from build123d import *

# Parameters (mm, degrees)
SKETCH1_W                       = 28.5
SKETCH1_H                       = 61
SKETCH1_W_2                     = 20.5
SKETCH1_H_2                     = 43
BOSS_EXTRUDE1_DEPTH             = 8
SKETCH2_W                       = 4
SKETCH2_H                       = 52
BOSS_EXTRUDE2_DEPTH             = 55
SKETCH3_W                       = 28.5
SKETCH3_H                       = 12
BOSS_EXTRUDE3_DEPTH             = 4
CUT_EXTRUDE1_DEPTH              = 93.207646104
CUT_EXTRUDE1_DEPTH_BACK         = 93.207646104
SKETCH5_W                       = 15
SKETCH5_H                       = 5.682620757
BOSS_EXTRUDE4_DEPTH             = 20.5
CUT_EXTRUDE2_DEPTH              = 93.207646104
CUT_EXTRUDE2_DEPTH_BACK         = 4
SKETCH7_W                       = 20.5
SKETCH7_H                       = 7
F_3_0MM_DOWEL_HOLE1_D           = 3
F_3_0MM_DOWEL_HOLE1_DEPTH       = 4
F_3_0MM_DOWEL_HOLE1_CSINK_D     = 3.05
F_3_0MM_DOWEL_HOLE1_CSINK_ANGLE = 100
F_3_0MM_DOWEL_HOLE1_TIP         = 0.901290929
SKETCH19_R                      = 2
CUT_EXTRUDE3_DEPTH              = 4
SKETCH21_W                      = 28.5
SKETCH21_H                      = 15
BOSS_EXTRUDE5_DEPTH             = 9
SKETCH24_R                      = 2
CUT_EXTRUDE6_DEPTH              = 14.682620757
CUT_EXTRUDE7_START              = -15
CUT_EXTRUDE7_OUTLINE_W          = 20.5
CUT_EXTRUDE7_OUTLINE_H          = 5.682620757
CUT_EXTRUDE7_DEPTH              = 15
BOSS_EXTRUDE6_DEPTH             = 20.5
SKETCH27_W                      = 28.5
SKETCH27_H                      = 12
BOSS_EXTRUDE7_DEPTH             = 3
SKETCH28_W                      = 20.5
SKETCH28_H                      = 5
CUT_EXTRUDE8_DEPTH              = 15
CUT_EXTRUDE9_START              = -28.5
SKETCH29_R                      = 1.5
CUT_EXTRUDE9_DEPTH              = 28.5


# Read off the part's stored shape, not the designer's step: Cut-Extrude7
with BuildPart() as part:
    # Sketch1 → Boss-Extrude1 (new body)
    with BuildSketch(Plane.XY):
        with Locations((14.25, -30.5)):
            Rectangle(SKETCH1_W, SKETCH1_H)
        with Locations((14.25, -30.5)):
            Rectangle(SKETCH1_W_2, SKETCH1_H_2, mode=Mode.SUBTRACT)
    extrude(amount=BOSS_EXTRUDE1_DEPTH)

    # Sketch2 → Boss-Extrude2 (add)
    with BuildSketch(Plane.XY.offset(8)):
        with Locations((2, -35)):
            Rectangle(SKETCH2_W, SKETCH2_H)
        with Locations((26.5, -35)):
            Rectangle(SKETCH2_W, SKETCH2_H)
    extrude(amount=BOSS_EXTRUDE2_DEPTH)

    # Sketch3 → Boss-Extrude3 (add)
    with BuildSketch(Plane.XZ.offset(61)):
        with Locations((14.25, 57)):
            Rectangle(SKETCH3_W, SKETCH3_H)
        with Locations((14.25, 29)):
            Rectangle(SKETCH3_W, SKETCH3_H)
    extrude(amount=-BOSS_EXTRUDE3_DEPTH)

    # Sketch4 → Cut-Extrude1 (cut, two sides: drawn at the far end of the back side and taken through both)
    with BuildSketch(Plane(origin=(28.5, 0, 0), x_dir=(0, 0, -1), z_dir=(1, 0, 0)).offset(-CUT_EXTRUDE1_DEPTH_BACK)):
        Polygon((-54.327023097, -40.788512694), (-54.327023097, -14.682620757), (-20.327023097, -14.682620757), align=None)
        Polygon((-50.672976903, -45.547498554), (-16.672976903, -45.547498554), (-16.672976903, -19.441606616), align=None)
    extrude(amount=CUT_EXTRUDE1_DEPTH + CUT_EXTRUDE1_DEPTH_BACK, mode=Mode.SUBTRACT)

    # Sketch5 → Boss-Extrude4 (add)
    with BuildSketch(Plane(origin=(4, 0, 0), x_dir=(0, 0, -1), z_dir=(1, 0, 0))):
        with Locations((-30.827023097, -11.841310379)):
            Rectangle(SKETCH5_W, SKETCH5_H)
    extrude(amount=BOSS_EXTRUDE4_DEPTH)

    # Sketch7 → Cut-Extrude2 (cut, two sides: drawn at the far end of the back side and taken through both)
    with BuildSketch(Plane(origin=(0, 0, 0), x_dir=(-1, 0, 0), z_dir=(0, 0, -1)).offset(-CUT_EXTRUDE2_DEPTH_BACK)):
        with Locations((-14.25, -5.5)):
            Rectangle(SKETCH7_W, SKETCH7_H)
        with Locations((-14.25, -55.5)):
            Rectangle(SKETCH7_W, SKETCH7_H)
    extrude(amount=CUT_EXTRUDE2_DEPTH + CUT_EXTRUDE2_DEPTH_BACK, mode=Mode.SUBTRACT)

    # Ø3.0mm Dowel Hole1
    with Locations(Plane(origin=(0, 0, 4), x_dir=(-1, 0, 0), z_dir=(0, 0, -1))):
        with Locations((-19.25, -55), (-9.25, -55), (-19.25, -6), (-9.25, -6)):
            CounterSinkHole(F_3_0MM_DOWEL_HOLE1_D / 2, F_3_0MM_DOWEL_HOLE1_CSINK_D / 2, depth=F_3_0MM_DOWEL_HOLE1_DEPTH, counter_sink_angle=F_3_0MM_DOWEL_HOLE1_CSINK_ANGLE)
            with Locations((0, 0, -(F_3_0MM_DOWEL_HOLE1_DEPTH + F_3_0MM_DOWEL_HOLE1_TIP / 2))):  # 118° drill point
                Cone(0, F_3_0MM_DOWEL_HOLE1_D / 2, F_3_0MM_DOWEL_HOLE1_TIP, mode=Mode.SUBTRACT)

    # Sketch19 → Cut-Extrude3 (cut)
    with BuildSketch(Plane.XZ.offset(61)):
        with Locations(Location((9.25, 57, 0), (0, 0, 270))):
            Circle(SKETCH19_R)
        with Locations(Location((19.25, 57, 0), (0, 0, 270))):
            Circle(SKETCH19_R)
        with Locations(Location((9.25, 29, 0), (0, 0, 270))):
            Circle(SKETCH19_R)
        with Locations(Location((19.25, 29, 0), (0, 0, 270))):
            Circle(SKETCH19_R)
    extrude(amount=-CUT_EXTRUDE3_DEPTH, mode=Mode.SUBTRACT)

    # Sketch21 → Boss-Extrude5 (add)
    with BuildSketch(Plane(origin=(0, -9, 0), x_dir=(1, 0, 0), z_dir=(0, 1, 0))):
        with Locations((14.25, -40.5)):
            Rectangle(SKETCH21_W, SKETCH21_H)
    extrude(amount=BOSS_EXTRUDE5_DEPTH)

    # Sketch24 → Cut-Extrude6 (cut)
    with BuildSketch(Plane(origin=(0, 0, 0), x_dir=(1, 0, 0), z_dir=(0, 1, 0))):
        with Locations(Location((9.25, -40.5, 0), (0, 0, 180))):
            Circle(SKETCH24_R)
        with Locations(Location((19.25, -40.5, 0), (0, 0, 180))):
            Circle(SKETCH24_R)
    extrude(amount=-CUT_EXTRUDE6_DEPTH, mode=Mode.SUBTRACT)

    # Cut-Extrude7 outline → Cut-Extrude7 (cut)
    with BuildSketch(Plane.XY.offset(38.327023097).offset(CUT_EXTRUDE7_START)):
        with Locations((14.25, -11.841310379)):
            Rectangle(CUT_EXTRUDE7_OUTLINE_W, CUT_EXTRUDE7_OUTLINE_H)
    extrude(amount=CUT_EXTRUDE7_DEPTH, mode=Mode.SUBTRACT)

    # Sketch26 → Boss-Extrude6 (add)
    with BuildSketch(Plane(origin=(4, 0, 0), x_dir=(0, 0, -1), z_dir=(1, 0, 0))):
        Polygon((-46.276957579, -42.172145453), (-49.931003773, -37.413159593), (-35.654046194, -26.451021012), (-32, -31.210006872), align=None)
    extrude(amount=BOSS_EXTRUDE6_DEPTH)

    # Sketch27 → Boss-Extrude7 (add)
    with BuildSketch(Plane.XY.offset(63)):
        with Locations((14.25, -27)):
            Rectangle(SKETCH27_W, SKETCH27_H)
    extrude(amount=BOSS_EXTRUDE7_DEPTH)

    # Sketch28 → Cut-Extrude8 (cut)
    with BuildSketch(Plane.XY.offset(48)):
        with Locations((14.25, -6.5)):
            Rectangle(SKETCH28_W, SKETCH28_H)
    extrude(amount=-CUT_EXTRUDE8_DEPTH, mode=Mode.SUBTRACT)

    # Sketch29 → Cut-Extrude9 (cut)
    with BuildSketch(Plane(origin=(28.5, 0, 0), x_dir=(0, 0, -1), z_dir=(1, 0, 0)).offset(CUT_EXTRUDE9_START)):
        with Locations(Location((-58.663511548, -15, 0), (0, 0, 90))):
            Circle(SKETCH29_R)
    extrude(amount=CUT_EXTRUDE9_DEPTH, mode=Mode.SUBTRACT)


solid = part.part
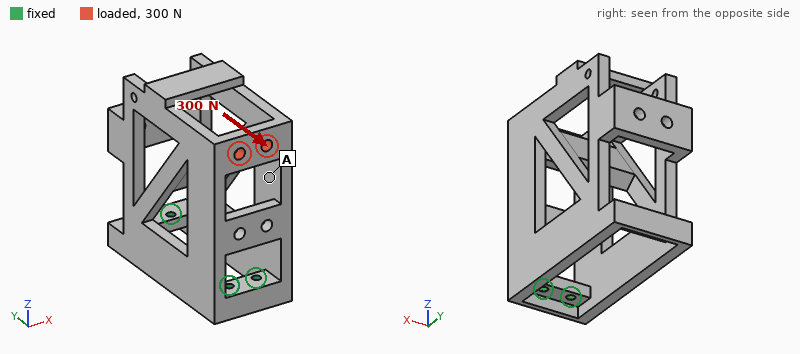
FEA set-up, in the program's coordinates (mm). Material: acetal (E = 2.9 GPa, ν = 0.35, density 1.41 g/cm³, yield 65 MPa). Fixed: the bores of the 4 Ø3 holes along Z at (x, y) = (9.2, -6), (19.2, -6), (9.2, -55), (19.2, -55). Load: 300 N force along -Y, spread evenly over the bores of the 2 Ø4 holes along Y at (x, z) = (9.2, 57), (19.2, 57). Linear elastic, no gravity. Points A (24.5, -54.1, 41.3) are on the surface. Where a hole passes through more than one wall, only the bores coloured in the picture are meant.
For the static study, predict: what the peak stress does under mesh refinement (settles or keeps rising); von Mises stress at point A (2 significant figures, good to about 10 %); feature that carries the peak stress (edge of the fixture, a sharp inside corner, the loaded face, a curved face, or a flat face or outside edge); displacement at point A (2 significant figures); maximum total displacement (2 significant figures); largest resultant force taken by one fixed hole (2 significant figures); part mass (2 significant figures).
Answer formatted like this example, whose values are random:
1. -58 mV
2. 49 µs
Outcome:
1. keeps rising
2. 4.1 MPa
3. edge of the fixture
4. 0.32 mm
5. 0.68 mm
6. 180 N
7. 40 g
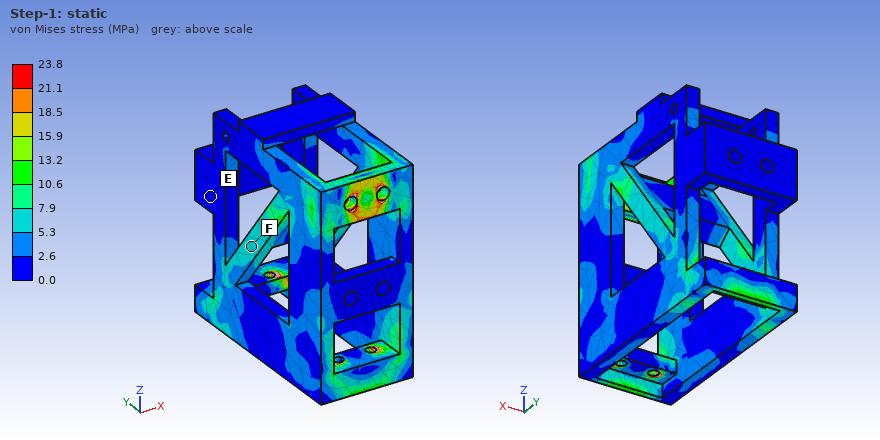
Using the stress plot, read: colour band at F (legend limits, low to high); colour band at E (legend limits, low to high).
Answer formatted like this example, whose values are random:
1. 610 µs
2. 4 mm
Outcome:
1. 5.3 to 7.9 MPa
2. 0.0 to 2.6 MPa
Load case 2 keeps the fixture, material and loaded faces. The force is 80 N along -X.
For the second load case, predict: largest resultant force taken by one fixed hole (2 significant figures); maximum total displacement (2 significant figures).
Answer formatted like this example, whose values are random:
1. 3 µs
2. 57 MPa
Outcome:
1. 140 N
2. 0.94 mm
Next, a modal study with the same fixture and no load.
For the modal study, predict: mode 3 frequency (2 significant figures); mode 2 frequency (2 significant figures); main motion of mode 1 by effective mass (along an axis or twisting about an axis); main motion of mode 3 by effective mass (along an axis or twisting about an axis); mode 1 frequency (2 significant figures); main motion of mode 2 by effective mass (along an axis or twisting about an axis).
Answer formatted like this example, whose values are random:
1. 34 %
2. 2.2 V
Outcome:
1. 970 Hz
2. 870 Hz
3. along X
4. along Y
5. 340 Hz
6. twisting about Z
